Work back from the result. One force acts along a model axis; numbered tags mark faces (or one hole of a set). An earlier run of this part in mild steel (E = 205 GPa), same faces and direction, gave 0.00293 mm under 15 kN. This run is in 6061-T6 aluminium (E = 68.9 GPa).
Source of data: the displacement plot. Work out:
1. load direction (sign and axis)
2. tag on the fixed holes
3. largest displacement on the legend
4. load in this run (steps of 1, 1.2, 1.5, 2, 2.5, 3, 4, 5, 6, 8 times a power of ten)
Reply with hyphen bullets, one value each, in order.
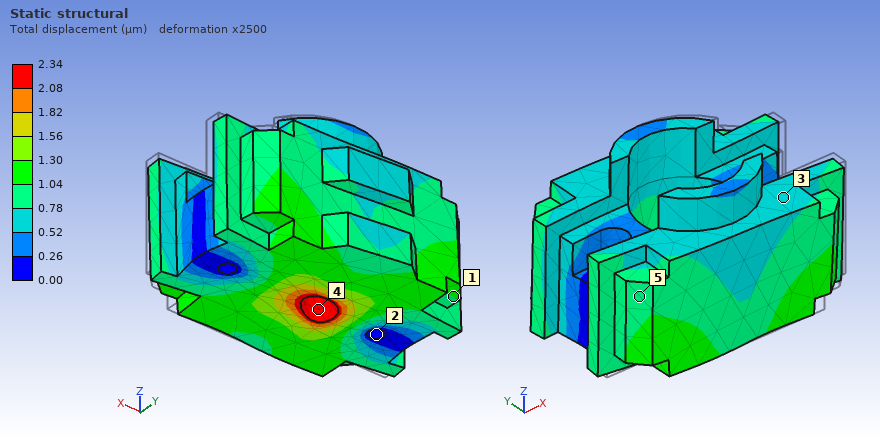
- -X
- 2
- 2.34 µm
- 4 kN
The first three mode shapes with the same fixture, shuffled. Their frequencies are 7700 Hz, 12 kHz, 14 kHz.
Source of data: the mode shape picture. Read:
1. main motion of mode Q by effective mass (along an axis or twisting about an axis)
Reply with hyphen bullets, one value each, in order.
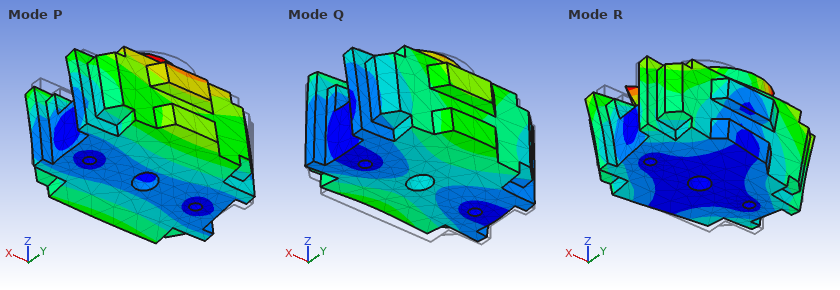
- along Z
